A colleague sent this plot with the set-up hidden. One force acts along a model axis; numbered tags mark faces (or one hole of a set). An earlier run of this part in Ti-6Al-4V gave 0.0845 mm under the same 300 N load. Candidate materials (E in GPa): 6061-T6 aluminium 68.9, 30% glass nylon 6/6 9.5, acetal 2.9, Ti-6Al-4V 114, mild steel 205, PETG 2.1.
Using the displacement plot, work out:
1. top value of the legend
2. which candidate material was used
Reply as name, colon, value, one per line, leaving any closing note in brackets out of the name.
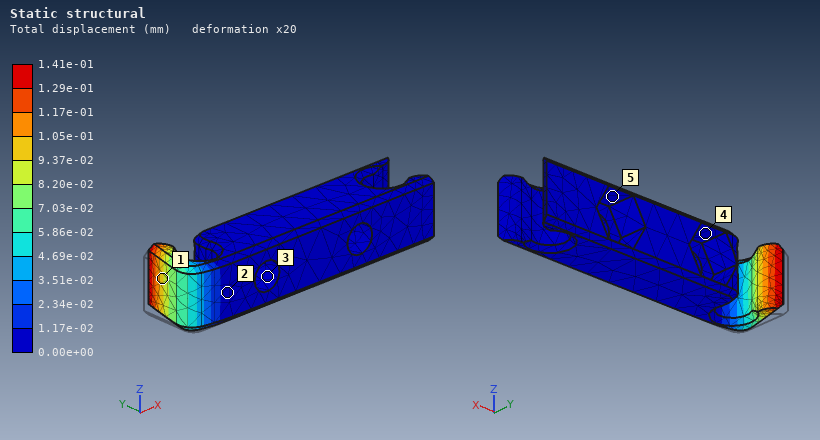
top value of the legend: 1.41e-01 mm
which candidate material was used: 6061-T6 aluminium
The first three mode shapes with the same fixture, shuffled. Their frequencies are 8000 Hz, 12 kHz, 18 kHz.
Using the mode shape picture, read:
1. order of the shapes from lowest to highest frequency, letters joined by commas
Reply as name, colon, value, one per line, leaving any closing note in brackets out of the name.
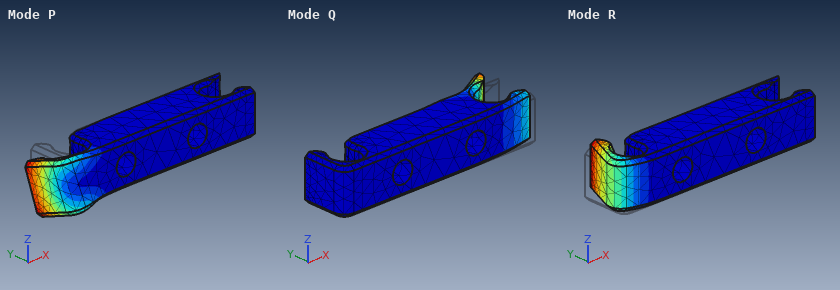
order of the shapes from lowest to highest frequency, letters joined by commas: R, P, Q
